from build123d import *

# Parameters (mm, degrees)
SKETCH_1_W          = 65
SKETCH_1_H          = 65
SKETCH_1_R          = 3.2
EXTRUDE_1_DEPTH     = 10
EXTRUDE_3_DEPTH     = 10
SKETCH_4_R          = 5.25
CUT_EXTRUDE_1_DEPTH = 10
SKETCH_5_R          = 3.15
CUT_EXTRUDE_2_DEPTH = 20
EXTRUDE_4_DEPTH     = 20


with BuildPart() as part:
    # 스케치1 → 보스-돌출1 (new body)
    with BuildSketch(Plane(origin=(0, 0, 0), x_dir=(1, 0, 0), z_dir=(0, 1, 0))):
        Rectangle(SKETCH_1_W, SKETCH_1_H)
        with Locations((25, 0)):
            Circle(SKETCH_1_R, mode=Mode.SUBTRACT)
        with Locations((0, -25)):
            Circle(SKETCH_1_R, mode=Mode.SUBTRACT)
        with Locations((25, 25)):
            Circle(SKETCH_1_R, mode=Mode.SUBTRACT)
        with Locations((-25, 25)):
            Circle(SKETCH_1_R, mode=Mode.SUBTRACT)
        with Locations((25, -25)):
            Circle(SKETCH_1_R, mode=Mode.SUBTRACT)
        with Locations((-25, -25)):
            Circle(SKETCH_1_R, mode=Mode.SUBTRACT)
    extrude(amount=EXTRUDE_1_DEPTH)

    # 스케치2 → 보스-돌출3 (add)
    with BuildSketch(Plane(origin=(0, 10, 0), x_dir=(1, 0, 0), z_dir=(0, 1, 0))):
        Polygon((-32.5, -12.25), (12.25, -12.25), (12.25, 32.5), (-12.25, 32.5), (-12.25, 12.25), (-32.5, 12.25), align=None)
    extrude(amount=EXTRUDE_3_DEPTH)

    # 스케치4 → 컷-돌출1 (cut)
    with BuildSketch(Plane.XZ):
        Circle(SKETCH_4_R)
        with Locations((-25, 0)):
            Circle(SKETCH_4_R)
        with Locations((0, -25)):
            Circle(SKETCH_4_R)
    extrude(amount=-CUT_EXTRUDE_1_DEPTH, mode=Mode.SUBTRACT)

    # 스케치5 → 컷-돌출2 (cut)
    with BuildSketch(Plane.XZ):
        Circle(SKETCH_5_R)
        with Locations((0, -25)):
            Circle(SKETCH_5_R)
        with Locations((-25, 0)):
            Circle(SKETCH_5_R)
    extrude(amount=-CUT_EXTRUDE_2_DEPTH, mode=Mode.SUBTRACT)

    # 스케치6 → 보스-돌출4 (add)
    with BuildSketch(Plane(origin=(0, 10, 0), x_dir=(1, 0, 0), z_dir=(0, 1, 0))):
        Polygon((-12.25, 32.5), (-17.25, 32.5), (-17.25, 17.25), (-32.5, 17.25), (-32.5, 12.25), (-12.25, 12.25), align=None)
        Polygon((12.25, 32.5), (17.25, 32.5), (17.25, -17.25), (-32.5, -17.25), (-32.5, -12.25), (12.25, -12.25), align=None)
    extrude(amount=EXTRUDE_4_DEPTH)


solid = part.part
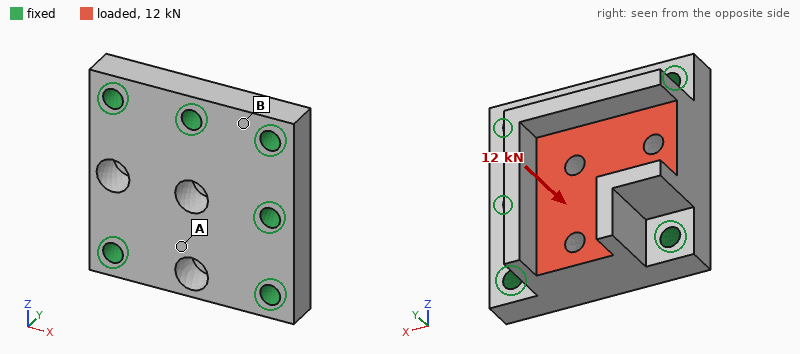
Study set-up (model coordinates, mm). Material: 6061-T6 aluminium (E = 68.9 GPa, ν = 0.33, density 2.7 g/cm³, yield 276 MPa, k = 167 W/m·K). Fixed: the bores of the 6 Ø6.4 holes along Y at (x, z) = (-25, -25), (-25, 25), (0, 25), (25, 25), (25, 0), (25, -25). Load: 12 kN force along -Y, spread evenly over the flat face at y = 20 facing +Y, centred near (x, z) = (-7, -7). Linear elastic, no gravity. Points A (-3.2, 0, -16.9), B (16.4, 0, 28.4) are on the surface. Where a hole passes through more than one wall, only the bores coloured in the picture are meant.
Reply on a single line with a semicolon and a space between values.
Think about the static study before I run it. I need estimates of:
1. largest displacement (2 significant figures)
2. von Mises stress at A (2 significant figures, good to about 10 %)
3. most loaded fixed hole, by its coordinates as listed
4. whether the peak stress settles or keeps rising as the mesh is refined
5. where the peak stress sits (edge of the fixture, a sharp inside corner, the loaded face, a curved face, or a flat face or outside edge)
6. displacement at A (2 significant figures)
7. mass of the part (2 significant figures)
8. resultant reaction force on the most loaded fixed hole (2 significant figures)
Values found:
14 µm; 16 MPa; (-25, -25); keeps rising; edge of the fixture; 12 µm; 180 g; 5.1 kN
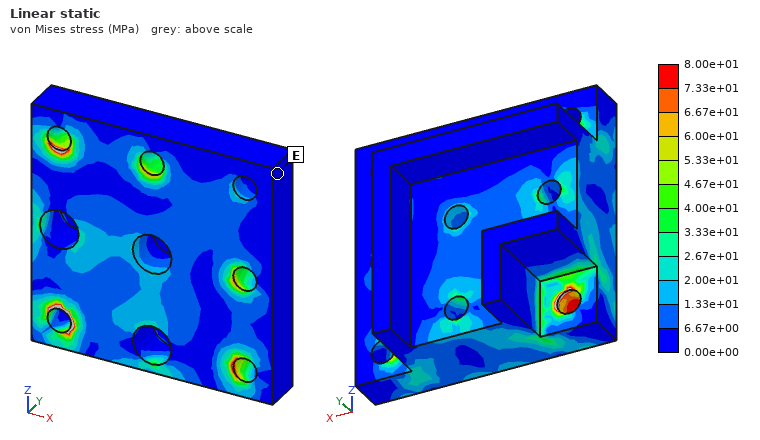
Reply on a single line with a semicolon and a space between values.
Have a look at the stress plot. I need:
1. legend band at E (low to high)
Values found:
0.00e+00 to 6.67e+00 MPa
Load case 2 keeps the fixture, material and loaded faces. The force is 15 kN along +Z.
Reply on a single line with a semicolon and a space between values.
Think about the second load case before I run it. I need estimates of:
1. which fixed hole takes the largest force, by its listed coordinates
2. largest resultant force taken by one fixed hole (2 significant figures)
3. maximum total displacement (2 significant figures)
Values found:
(-25, -25); 4.9 kN; 24 µm
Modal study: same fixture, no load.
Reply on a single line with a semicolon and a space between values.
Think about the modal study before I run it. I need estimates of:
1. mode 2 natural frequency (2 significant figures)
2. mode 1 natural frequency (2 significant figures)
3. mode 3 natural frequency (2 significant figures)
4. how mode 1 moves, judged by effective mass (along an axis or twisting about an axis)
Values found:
17 kHz; 15 kHz; 20 kHz; along Y
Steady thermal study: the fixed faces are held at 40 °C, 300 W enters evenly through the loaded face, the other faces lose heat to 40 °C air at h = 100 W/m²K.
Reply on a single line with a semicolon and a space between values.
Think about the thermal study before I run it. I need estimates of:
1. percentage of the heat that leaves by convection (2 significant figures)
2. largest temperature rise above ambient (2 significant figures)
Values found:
7.2 %; 33 K
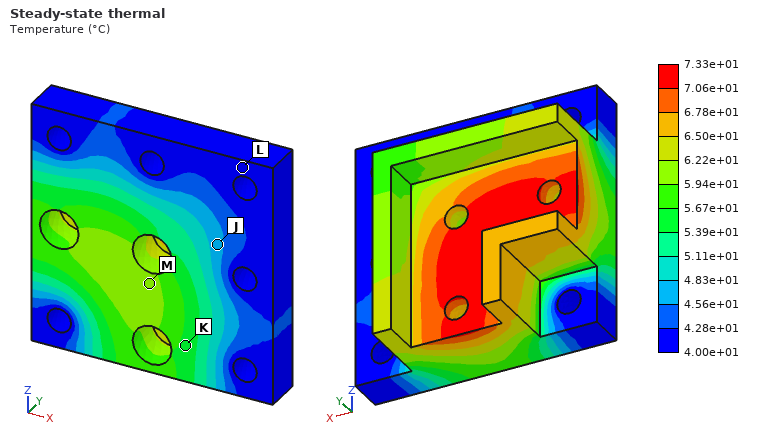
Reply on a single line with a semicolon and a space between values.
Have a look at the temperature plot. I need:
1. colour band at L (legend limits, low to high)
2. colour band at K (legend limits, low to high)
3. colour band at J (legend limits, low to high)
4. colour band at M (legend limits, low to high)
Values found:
4.00e+01 to 4.28e+01 °C; 5.39e+01 to 5.67e+01 °C; 4.56e+01 to 4.83e+01 °C; 5.94e+01 to 6.22e+01 °C
